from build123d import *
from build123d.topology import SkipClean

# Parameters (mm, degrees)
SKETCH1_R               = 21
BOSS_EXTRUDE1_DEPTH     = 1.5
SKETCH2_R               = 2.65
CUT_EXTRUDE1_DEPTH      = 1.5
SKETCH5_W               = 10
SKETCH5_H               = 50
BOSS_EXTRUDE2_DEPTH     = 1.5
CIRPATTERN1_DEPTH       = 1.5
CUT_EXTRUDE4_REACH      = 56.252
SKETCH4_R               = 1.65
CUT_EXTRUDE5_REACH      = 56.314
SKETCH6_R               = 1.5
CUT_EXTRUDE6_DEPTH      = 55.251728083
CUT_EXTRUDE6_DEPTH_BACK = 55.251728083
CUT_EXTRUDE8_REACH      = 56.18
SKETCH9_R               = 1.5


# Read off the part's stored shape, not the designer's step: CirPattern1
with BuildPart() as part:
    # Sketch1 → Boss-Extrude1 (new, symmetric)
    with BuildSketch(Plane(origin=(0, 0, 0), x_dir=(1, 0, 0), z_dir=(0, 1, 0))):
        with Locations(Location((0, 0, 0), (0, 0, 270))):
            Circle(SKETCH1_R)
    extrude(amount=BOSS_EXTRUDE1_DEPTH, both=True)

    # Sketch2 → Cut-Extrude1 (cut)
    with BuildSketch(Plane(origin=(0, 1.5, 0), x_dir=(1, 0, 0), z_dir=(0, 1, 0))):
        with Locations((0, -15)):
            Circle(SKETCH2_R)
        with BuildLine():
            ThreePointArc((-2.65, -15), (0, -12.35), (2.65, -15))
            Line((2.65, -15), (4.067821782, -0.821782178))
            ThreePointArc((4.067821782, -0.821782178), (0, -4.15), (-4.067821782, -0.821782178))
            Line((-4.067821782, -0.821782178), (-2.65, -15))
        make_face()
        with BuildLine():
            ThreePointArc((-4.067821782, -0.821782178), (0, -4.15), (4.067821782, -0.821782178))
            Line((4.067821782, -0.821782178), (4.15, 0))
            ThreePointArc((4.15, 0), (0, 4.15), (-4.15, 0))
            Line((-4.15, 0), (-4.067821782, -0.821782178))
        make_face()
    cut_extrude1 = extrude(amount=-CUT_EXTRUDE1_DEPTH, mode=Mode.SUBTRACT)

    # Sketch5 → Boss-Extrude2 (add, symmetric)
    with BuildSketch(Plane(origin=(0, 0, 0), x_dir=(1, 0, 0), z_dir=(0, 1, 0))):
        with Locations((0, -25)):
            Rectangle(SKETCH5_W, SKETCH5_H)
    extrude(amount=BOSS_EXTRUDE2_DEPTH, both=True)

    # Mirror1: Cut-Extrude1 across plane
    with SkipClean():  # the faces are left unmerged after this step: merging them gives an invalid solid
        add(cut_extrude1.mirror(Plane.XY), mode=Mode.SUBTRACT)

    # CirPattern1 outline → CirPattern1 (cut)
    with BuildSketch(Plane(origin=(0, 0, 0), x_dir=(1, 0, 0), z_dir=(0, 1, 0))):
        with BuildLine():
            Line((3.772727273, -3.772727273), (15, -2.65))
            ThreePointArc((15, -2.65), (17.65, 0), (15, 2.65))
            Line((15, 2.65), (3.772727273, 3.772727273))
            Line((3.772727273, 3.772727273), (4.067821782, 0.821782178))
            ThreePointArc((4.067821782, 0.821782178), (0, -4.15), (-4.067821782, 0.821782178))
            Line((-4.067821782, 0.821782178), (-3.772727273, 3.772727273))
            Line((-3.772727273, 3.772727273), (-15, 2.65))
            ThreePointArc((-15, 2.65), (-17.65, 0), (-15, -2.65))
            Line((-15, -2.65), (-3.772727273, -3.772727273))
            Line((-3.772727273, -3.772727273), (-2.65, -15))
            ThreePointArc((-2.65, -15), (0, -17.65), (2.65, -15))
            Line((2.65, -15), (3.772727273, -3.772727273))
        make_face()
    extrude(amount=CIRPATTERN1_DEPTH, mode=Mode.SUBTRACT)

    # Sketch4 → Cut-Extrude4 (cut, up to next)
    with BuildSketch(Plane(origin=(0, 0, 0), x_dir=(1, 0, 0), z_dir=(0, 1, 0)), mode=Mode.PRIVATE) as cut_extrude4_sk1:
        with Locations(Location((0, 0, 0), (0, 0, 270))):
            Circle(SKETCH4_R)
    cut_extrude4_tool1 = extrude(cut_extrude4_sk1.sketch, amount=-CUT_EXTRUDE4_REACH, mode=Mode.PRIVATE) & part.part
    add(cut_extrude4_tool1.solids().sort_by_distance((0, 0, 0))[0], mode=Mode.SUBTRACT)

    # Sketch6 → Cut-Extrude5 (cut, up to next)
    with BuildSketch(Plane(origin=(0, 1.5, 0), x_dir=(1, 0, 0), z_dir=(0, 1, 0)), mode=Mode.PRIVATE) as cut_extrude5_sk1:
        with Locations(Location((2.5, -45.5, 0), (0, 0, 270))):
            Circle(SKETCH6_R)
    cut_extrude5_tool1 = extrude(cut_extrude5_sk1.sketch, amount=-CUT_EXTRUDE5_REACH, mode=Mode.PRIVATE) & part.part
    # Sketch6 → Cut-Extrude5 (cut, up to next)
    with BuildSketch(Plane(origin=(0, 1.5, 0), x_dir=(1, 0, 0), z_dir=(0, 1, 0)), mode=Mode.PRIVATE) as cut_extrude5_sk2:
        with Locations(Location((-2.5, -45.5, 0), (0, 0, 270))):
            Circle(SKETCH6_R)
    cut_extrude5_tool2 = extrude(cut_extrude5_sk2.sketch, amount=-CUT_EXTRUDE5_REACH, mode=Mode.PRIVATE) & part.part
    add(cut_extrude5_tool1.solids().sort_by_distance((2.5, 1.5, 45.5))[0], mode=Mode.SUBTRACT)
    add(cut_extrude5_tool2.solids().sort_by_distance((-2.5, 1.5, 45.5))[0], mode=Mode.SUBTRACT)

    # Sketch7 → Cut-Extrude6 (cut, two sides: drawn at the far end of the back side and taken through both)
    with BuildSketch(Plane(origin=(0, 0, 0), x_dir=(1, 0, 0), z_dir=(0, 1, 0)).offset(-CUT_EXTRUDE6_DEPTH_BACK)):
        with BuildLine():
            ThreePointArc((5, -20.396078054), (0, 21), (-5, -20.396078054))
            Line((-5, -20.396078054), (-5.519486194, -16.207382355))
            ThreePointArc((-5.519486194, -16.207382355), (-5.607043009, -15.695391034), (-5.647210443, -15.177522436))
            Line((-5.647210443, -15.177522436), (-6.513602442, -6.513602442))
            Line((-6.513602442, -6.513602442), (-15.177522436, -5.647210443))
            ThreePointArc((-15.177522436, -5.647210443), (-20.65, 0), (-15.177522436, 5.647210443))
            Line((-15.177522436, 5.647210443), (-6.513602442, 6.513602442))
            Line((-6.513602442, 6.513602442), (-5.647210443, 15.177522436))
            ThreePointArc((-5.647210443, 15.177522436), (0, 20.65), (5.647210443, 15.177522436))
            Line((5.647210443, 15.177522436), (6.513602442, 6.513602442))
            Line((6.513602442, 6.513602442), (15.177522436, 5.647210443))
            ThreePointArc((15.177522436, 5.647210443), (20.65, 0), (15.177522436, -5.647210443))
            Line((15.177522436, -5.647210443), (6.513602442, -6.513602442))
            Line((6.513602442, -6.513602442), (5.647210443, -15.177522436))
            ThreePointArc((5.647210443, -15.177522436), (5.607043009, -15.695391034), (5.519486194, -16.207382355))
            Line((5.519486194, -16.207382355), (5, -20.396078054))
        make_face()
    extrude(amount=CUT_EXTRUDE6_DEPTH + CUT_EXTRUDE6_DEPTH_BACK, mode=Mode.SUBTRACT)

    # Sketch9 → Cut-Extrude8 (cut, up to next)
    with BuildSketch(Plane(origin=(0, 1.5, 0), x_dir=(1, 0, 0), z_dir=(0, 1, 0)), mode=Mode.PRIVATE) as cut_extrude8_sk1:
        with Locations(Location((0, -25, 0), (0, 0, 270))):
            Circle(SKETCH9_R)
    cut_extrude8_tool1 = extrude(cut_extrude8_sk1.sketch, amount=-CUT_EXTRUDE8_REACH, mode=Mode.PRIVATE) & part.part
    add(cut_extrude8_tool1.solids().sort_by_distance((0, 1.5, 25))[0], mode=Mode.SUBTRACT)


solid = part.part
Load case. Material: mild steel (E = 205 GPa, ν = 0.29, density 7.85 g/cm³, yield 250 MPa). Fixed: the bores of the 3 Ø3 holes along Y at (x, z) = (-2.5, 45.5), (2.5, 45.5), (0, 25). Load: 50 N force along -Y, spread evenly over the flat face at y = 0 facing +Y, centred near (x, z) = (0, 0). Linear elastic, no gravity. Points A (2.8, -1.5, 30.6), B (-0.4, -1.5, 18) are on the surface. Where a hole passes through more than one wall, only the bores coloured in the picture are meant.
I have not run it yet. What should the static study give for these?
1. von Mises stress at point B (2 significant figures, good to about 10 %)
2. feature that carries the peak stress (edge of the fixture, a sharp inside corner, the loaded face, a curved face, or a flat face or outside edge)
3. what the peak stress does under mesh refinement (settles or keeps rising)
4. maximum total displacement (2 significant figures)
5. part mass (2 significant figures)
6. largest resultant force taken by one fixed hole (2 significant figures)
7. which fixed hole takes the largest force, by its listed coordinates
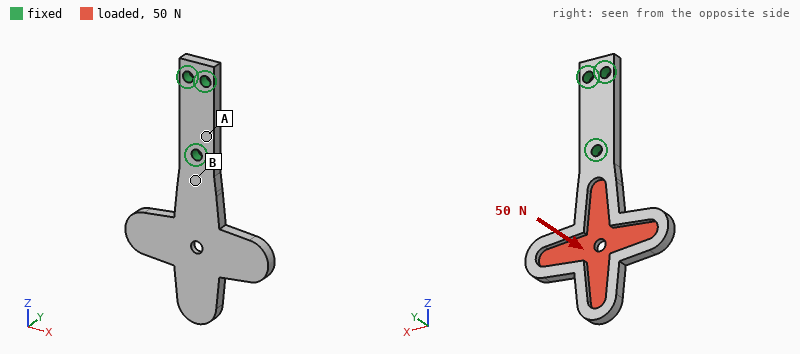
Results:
60 MPa
edge of the fixture
keeps rising
0.15 mm
20 g
54 N
(0, 25)
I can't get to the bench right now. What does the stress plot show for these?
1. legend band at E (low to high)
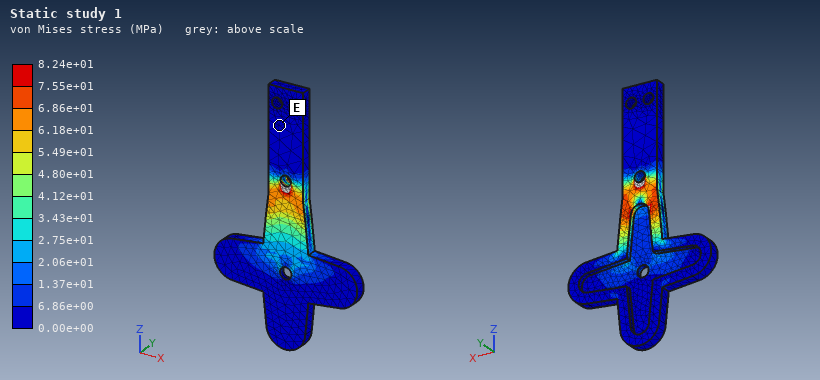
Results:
0.00e+00 to 6.86e+00 MPa
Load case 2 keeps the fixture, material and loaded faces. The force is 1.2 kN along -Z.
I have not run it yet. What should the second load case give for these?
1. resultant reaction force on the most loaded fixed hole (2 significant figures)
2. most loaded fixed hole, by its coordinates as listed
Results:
1.1 kN
(0, 25)
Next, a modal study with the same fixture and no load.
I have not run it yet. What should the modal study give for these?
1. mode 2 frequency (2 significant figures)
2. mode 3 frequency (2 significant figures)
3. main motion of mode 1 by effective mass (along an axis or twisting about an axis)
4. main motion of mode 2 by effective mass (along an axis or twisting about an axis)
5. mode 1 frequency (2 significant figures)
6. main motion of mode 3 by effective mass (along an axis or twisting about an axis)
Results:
1900 Hz
2900 Hz
along Y
twisting about Z
1000 Hz
along X
